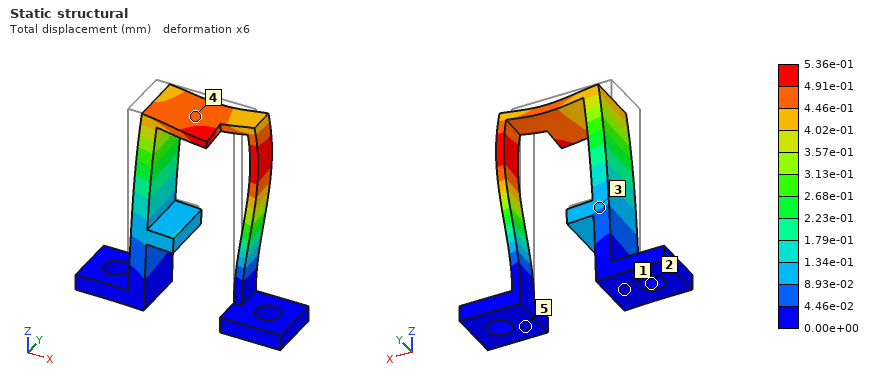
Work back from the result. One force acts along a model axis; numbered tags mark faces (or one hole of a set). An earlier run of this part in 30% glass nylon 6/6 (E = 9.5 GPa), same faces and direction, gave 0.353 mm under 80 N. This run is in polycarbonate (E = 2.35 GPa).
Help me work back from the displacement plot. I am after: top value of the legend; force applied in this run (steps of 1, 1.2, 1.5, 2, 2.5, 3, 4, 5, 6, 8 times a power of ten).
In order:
5.36e-01 mm
30 N
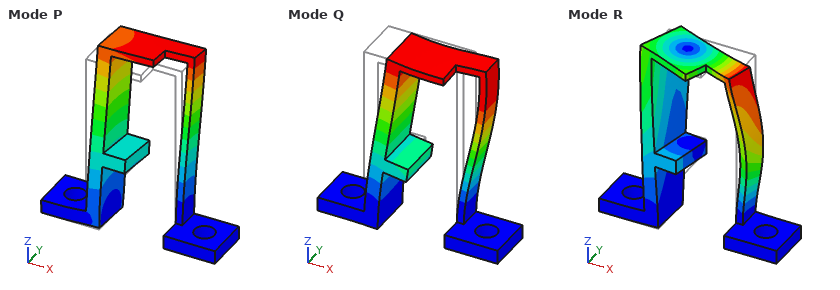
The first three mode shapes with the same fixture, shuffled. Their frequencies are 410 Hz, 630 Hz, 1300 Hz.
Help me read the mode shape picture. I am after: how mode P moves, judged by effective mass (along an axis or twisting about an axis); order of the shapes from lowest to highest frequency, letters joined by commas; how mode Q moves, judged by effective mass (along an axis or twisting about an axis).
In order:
along Y
Q, P, R
along X
